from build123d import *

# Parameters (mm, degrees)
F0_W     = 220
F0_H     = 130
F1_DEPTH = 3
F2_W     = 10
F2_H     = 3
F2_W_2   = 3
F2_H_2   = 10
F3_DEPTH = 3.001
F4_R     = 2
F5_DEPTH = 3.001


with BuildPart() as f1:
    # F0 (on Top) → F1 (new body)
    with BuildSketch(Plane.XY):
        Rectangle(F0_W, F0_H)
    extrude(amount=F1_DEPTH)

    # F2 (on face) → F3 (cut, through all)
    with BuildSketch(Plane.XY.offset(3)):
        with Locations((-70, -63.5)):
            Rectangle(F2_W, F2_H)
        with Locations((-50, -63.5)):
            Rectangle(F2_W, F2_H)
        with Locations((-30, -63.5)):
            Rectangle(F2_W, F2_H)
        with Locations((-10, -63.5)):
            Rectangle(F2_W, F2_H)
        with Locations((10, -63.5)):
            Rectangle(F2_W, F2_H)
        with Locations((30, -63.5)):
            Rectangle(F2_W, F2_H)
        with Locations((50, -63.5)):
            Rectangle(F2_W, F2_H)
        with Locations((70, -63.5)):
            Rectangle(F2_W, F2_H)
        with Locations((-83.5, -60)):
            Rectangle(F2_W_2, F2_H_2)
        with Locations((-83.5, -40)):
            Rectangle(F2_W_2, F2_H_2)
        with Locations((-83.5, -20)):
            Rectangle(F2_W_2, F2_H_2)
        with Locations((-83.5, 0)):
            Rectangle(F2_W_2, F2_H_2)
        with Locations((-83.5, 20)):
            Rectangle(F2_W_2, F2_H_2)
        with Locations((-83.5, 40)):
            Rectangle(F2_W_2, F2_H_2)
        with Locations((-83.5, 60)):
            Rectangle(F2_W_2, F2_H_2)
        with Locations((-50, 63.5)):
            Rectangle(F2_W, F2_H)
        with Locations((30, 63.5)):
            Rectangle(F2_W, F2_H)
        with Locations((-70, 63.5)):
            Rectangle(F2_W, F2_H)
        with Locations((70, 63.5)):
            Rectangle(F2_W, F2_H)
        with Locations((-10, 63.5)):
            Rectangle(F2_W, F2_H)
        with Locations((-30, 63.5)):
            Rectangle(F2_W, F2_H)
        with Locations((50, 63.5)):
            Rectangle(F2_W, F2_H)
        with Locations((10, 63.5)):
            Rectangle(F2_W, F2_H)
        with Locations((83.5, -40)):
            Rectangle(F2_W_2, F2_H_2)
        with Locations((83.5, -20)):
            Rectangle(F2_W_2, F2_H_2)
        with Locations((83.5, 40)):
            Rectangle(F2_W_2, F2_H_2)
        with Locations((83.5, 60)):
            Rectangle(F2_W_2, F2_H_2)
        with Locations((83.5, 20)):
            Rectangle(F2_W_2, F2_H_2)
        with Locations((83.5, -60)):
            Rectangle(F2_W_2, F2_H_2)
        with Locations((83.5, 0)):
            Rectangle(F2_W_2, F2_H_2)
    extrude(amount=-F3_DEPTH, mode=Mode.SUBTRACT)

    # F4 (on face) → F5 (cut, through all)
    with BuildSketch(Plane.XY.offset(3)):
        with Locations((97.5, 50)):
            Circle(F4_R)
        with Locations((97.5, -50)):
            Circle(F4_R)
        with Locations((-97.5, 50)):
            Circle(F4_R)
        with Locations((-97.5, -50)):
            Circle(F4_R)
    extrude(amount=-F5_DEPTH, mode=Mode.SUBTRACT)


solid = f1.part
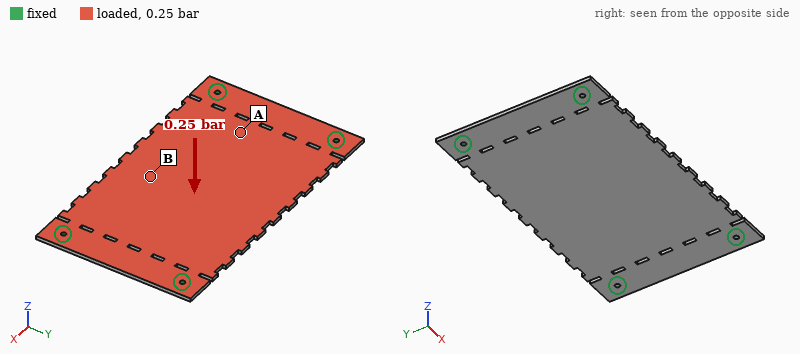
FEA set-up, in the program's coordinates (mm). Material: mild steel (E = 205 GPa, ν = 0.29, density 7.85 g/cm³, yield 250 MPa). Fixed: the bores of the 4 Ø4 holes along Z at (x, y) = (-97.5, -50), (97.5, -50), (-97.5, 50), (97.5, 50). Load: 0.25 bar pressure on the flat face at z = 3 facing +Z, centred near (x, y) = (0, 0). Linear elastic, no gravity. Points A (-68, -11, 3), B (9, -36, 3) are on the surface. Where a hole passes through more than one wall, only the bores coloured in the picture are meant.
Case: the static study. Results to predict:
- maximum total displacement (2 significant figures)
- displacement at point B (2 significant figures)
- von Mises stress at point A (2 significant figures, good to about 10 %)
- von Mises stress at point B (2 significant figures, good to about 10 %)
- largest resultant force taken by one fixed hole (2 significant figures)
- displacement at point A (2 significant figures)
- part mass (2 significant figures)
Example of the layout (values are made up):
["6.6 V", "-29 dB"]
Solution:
["0.32 mm", "0.31 mm", "12 MPa", "32 MPa", "170 N", "0.13 mm", "650 g"]
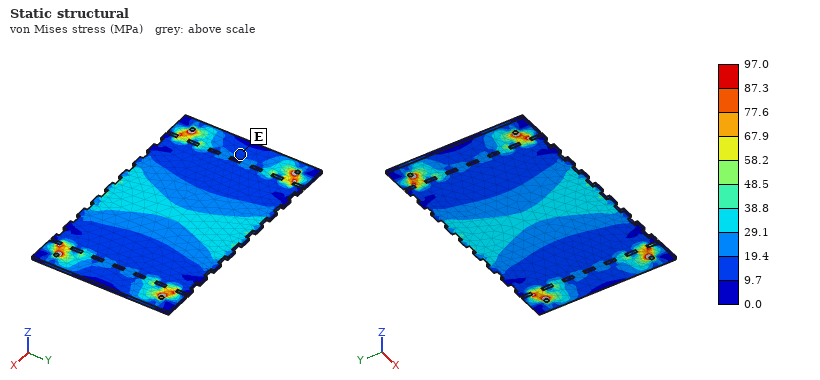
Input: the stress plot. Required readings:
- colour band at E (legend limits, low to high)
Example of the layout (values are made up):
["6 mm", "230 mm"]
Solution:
["9.7 to 19.4 MPa"]
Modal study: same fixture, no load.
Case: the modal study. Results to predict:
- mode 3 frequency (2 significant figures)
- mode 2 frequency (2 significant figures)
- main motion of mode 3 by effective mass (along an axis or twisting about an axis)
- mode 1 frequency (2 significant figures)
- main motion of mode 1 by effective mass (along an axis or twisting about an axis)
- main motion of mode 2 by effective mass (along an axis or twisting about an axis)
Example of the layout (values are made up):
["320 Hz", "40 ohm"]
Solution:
["940 Hz", "550 Hz", "twisting about Y", "330 Hz", "along Z", "twisting about X"]
